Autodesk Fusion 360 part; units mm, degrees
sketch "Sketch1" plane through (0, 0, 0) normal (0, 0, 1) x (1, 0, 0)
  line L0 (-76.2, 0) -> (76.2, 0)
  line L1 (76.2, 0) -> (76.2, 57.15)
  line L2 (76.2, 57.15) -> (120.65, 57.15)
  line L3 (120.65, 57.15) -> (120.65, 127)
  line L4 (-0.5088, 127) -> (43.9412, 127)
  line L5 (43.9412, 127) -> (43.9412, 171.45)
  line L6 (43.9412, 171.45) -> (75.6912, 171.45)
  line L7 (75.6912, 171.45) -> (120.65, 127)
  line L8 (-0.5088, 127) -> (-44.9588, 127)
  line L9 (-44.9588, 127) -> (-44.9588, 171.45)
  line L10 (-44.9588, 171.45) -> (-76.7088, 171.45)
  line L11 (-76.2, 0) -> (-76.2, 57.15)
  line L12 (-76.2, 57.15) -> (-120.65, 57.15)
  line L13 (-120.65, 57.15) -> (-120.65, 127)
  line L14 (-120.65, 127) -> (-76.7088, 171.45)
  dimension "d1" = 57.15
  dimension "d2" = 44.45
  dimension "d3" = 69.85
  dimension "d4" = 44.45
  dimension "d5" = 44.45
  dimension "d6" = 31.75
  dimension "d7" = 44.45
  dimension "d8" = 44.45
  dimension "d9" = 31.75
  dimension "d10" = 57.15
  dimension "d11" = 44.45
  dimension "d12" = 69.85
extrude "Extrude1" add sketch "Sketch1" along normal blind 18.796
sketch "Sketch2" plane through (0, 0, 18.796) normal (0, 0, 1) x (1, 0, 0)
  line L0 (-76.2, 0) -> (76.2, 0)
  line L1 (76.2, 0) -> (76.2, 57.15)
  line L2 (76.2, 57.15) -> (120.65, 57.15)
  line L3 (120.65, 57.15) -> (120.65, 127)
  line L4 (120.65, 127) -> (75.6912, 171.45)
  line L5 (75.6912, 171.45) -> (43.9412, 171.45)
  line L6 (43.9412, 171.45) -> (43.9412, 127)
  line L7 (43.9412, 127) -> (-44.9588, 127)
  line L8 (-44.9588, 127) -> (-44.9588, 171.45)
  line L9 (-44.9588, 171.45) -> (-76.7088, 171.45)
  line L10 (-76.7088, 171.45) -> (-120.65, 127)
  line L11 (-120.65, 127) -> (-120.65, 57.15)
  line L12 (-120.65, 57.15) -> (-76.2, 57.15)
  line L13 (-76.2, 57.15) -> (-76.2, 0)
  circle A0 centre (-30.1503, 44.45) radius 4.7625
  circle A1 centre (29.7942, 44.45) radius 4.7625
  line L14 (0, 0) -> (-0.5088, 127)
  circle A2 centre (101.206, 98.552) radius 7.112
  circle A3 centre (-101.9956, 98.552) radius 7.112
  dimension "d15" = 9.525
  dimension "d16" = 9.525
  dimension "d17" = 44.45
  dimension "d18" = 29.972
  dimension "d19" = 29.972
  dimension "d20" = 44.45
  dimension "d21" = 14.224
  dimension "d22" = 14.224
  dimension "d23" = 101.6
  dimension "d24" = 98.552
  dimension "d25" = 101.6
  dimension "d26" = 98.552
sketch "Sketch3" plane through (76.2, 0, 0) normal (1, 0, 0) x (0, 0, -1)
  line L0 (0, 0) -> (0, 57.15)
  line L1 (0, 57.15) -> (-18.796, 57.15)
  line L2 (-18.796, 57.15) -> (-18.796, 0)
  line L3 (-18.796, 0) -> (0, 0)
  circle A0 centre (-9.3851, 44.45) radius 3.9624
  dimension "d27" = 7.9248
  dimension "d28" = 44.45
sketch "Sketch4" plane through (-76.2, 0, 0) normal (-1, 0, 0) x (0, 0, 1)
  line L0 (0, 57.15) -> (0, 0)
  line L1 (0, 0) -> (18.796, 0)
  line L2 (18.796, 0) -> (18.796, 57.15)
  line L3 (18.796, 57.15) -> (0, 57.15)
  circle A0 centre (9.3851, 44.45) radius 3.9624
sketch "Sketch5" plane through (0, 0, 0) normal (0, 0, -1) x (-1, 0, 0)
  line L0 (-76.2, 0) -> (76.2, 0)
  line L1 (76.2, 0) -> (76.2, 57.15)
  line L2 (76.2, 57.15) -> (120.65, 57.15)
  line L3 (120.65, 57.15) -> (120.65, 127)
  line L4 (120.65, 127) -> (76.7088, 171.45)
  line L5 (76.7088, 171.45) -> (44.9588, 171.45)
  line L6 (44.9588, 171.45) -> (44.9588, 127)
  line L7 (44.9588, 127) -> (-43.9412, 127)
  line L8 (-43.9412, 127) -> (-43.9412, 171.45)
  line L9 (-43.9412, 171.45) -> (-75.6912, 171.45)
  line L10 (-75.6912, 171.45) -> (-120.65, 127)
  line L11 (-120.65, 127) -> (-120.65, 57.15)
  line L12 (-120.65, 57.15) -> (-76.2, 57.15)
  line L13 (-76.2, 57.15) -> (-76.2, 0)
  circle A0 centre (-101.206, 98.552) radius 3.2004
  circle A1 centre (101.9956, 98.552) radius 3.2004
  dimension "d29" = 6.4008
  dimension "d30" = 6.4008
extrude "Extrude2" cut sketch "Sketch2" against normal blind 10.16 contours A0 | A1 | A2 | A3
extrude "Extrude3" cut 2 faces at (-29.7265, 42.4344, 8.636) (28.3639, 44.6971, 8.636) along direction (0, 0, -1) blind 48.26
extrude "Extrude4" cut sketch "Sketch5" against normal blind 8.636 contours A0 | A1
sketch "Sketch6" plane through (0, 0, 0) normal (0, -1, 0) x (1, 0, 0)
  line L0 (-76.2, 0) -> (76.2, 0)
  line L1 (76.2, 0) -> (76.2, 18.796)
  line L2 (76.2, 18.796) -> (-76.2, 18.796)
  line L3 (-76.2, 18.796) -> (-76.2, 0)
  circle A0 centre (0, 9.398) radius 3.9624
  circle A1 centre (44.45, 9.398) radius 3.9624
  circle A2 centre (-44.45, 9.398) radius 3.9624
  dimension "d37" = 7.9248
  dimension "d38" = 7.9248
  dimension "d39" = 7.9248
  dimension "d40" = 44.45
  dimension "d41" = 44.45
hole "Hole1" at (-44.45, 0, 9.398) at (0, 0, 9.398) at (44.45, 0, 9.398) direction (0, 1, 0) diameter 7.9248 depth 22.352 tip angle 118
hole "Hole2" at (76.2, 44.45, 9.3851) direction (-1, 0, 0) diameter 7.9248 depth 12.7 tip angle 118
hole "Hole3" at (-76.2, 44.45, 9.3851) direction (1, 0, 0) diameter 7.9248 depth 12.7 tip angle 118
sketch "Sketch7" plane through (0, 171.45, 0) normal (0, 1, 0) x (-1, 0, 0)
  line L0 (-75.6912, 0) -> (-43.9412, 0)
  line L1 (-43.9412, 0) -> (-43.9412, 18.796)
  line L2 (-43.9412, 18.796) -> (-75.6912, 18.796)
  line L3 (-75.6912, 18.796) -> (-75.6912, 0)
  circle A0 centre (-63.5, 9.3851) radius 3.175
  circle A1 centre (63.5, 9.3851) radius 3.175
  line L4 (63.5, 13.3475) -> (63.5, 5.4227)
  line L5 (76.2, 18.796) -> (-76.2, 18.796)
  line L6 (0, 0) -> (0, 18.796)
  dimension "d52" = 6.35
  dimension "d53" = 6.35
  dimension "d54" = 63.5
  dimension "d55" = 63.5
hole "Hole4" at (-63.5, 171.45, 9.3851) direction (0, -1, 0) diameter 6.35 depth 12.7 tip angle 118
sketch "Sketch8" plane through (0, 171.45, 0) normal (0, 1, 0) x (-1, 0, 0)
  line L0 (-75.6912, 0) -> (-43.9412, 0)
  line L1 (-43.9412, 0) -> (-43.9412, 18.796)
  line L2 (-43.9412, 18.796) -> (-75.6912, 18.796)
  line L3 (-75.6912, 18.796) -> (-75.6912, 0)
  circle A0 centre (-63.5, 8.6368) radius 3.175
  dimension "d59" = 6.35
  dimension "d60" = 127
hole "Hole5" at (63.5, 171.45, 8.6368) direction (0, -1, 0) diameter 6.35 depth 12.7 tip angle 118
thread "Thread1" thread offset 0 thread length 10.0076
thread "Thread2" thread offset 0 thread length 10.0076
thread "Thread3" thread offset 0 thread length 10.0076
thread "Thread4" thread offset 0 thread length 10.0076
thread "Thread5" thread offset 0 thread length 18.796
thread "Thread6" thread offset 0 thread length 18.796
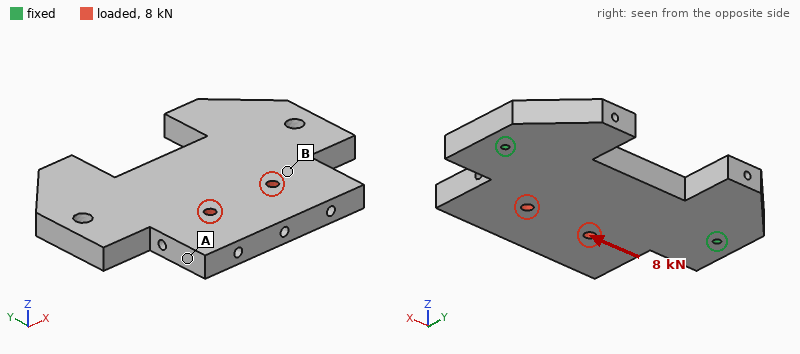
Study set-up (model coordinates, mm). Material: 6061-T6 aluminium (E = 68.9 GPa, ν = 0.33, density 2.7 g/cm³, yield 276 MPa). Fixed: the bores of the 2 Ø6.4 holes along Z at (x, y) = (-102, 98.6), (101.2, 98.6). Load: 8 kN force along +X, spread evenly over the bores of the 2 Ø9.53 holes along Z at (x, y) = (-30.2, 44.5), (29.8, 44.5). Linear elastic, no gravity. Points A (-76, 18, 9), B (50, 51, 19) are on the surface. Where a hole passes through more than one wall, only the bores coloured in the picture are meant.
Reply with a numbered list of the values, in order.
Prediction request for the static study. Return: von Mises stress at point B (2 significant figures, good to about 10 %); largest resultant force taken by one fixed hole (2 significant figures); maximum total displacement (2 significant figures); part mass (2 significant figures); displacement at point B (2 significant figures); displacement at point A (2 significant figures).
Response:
1. 4.7 MPa
2. 4.5 kN
3. 17 µm
4. 1.5 kg
5. 10 µm
6. 15 µm
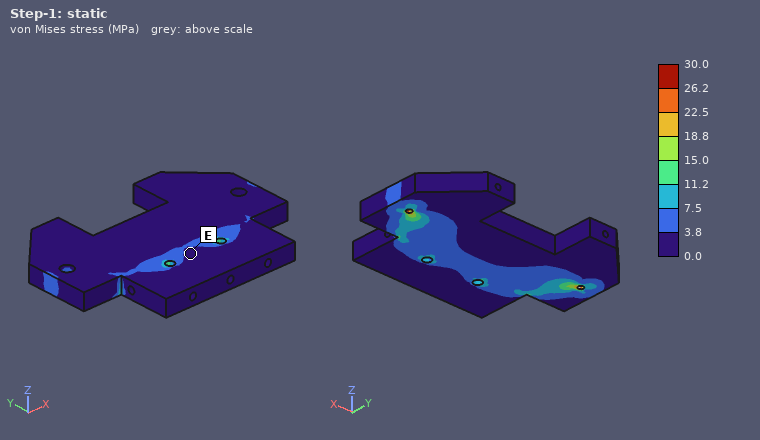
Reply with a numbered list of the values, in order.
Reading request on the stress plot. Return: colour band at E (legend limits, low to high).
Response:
1. 0.0 to 3.8 MPa
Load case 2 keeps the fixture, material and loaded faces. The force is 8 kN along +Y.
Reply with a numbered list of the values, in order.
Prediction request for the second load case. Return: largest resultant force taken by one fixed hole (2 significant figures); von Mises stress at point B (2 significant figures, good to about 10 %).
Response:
1. 4.3 kN
2. 5.4 MPa
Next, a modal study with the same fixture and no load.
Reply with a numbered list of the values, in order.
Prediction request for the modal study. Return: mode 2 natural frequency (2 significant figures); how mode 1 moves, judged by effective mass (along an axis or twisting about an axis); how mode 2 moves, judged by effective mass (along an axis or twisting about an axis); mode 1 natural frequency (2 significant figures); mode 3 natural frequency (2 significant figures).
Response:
1. 1300 Hz
2. along Z
3. along Z
4. 570 Hz
5. 1900 Hz
